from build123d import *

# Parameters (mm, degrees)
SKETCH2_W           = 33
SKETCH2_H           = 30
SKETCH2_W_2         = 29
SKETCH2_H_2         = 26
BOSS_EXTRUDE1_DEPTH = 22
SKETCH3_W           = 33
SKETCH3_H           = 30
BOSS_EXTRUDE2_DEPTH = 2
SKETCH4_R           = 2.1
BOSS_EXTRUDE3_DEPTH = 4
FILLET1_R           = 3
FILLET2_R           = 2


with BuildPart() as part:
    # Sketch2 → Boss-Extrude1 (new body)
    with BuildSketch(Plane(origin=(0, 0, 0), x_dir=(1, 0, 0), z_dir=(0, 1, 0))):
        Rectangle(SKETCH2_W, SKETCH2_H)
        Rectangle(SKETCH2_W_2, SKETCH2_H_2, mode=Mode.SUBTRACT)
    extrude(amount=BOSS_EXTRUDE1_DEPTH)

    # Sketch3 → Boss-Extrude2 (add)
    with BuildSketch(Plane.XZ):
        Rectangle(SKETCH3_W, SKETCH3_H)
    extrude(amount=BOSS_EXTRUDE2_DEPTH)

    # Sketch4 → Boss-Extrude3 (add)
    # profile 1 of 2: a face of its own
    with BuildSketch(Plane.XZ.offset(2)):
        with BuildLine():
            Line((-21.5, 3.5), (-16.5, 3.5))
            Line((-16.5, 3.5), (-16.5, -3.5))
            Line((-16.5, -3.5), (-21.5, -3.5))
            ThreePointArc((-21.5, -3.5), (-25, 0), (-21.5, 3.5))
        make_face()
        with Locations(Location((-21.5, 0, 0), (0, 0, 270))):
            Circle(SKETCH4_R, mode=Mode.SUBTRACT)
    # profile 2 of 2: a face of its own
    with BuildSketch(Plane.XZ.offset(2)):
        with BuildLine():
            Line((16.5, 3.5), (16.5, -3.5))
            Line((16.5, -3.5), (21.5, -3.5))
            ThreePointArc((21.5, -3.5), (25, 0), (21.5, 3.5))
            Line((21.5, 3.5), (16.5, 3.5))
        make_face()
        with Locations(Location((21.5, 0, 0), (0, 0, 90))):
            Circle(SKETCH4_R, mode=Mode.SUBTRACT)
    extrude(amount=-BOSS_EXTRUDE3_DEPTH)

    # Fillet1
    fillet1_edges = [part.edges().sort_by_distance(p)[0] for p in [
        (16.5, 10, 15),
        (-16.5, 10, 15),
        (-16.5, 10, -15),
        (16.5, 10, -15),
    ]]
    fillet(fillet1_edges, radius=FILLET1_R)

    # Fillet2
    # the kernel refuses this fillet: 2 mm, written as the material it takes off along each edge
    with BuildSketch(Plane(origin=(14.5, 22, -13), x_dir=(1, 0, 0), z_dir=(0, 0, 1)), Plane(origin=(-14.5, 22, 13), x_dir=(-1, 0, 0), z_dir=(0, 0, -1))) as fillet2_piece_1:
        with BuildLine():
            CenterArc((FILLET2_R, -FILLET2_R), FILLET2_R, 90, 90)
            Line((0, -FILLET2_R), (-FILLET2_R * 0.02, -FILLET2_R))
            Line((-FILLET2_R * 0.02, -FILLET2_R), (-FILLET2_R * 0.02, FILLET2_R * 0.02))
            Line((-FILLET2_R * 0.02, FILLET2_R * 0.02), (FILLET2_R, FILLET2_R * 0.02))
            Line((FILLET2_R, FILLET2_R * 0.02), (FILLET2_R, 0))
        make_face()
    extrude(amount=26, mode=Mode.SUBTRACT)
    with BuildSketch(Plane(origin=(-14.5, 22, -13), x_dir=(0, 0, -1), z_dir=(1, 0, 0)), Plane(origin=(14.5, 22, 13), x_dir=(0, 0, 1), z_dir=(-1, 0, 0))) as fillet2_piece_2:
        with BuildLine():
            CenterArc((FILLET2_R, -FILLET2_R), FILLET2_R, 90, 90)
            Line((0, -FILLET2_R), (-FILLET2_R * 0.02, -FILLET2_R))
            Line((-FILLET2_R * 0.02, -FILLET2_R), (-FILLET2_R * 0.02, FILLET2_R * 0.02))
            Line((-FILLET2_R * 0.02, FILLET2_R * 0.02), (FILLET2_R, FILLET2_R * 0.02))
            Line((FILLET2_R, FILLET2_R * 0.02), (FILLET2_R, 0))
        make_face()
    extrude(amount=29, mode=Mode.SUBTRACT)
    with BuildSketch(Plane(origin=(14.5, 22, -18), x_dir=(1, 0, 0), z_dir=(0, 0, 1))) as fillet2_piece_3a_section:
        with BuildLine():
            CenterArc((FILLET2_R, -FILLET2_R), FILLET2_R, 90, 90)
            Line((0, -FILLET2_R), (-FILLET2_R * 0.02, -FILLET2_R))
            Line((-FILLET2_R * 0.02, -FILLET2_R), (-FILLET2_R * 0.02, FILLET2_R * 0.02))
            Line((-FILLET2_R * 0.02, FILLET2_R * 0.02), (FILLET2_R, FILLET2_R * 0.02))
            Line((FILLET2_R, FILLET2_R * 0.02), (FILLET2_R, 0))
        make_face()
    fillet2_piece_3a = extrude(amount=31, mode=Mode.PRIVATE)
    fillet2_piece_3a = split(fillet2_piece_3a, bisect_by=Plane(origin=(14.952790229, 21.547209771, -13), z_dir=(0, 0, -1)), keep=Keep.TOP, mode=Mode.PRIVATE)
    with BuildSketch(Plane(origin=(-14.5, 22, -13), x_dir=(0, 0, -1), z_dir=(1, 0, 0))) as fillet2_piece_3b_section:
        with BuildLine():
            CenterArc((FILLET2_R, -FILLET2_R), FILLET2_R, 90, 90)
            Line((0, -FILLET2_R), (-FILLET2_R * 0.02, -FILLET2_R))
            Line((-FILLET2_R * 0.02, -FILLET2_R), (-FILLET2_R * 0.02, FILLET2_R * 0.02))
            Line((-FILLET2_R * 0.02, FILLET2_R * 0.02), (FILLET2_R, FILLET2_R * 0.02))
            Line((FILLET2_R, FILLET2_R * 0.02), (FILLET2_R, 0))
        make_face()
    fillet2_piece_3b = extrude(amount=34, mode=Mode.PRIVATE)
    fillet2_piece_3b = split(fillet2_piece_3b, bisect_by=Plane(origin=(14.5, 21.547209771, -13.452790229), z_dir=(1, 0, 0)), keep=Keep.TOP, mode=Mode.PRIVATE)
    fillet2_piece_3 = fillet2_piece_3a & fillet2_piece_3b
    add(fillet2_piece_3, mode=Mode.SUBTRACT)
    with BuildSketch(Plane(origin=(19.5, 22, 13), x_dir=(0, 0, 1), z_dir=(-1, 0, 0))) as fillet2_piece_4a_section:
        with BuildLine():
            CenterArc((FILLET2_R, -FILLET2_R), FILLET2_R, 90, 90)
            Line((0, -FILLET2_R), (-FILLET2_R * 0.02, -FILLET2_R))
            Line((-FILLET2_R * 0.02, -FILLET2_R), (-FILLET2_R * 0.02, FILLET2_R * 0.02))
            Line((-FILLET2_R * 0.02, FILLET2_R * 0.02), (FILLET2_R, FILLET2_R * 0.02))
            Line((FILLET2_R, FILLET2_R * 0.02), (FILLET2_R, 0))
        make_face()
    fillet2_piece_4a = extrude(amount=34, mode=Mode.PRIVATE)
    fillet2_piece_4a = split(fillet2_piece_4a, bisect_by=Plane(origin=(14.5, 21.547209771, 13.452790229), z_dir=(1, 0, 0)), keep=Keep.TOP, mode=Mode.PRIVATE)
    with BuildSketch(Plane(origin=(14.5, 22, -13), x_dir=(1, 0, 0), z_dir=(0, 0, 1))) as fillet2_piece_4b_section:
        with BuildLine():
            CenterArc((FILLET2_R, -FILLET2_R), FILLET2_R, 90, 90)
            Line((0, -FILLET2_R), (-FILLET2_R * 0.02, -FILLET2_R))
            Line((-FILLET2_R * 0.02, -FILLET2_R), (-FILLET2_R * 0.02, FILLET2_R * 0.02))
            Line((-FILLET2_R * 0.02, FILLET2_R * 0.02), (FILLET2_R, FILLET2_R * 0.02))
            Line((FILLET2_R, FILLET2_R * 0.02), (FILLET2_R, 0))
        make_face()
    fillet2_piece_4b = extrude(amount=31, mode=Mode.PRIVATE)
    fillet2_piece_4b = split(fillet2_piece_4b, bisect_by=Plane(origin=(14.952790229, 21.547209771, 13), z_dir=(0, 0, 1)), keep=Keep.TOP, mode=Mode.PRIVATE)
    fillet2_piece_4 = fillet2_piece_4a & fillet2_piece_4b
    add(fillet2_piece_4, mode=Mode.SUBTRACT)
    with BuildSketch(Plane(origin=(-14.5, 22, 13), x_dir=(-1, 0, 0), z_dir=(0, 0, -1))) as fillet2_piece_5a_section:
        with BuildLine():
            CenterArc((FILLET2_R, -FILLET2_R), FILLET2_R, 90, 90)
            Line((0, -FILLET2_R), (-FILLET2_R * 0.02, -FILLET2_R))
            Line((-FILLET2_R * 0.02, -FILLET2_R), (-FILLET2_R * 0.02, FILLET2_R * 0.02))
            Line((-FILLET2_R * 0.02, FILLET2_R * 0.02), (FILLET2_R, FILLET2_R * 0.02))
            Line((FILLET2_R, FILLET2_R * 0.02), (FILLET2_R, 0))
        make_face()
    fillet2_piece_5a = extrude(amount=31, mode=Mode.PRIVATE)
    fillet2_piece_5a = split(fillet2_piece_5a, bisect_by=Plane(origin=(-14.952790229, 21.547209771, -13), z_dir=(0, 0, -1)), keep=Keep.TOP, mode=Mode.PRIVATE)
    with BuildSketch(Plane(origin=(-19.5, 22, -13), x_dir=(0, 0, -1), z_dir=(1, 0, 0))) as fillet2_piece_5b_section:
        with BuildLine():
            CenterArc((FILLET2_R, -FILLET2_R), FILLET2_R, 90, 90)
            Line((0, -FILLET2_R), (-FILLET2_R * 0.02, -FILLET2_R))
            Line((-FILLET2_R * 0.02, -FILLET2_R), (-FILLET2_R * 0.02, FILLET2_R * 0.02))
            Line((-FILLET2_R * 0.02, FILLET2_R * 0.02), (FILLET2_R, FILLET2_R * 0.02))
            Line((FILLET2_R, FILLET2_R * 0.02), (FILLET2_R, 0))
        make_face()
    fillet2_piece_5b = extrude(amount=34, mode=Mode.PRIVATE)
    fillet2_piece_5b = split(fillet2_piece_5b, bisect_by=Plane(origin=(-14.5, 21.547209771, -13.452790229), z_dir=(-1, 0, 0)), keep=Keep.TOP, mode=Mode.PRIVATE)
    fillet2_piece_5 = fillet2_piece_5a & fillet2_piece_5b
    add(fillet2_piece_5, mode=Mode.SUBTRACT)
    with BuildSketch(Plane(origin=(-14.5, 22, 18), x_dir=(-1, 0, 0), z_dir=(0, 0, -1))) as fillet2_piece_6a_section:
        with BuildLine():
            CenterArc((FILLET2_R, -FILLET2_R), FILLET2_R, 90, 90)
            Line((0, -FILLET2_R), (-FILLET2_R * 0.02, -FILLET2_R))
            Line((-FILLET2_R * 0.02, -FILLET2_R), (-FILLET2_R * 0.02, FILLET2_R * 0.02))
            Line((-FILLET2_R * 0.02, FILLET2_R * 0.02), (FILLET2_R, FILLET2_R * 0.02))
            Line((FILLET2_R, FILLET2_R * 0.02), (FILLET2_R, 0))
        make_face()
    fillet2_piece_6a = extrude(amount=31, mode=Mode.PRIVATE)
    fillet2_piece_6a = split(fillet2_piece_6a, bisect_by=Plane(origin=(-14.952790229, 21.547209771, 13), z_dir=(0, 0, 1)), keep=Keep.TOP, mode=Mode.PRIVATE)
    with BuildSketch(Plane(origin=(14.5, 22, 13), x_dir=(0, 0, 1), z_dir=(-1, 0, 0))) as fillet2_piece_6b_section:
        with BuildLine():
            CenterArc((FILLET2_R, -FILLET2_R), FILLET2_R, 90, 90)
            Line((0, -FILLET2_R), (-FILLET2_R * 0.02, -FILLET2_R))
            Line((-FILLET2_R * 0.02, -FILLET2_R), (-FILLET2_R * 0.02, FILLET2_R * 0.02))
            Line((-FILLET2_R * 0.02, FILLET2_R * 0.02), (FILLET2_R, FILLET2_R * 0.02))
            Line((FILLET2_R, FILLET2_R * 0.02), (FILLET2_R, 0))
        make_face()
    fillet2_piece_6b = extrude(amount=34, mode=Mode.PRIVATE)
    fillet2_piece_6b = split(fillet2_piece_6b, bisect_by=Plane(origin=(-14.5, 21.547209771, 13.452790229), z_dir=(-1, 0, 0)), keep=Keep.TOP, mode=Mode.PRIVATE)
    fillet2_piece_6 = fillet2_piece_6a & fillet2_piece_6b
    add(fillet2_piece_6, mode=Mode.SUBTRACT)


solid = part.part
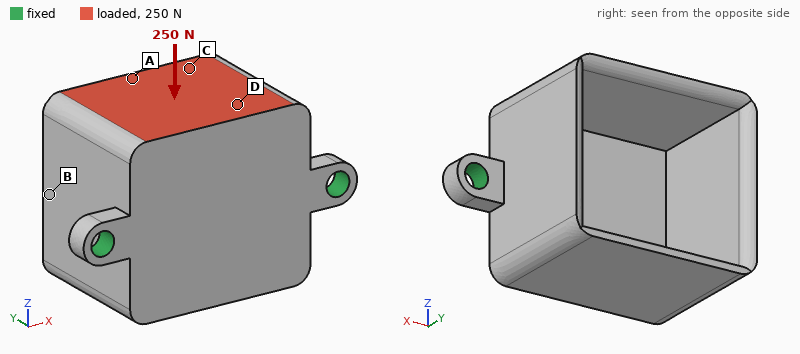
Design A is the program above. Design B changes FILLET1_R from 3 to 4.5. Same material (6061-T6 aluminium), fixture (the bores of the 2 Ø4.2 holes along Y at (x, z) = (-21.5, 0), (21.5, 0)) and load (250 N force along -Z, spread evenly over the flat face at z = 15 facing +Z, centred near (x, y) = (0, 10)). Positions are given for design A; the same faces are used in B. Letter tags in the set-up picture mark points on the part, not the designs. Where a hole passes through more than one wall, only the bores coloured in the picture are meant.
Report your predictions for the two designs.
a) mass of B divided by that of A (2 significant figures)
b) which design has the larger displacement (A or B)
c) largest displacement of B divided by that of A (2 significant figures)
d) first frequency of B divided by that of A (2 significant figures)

0.97
B
1.1
1.0
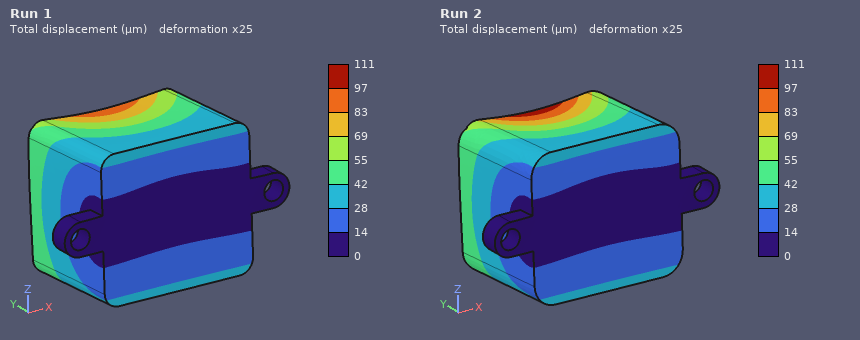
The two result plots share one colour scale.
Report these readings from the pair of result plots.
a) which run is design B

Run 2
